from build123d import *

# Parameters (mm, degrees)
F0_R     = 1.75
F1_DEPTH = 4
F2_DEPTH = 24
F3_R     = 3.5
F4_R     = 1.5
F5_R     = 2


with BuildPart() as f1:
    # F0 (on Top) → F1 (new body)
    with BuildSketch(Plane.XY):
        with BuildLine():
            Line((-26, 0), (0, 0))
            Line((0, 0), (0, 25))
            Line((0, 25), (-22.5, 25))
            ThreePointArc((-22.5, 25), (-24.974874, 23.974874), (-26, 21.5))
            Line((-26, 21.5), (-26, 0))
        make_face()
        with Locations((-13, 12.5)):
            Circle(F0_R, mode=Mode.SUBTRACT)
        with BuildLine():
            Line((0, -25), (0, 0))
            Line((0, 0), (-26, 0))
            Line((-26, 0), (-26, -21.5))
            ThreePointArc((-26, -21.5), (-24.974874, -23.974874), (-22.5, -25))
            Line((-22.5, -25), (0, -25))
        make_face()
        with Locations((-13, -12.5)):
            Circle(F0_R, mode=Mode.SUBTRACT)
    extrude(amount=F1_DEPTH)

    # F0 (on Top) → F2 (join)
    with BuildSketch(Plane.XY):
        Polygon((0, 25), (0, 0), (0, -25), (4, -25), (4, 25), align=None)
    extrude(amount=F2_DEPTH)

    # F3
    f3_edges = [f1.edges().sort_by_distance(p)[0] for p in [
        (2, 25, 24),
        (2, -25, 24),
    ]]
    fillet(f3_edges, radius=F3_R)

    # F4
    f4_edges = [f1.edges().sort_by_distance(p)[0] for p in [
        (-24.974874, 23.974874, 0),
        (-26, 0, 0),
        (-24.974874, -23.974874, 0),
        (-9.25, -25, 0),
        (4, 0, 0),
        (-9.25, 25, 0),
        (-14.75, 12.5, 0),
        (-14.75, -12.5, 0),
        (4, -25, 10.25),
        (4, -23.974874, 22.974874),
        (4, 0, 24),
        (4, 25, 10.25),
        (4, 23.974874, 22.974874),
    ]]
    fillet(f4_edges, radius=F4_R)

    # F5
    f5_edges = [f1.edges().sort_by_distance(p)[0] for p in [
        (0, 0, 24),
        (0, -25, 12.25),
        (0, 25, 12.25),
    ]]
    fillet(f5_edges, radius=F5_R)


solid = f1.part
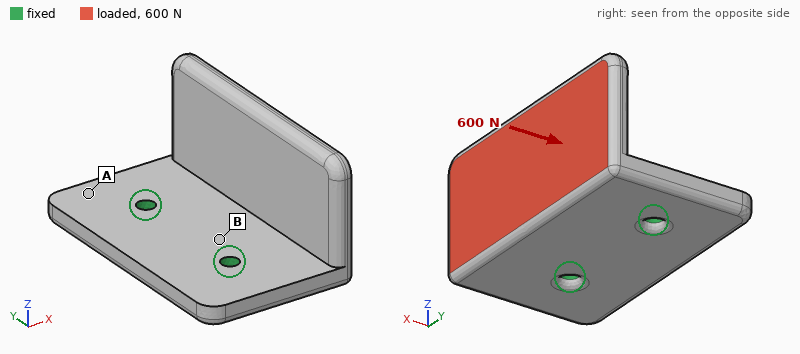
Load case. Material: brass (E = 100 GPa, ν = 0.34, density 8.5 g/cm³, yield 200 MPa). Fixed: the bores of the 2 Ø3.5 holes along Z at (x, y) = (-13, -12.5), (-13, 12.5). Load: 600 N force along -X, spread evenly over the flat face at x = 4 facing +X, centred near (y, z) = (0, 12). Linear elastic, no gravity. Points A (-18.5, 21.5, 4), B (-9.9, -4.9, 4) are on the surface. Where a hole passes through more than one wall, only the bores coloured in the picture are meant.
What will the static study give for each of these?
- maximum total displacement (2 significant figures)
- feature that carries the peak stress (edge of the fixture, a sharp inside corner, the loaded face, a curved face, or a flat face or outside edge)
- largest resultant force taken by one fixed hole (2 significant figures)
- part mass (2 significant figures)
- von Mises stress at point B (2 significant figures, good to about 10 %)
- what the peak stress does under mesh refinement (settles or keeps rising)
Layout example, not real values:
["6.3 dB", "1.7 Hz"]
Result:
["0.11 mm", "edge of the fixture", "300 N", "82 g", "35 MPa", "keeps rising"]
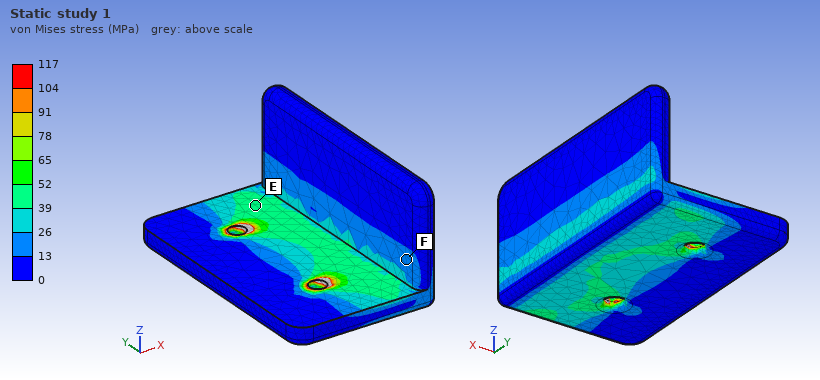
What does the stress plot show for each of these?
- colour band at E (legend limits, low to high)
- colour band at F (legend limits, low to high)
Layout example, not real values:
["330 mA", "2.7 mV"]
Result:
["39 to 52 MPa", "13 to 26 MPa"]
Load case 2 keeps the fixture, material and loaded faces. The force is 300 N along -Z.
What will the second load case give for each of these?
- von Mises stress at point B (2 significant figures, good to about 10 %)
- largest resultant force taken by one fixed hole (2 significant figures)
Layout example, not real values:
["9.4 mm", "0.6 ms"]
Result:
["22 MPa", "150 N"]
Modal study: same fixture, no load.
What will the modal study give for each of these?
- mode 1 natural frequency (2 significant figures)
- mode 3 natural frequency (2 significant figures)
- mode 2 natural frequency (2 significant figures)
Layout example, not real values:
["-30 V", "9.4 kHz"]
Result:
["1900 Hz", "5200 Hz", "3100 Hz"]
